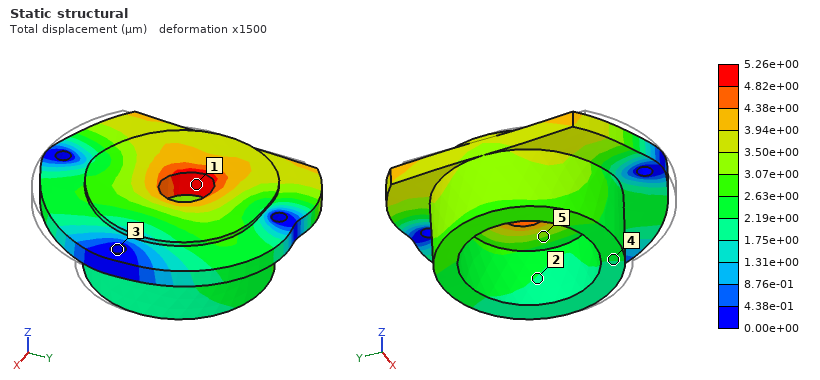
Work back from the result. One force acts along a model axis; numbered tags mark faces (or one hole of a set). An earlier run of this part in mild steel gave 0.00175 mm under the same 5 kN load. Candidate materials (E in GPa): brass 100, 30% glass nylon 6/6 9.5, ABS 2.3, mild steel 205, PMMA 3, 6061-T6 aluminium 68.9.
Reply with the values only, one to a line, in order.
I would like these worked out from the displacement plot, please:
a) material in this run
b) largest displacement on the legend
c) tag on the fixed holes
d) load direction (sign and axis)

6061-T6 aluminium
5.26e+00 µm
3
+Y
